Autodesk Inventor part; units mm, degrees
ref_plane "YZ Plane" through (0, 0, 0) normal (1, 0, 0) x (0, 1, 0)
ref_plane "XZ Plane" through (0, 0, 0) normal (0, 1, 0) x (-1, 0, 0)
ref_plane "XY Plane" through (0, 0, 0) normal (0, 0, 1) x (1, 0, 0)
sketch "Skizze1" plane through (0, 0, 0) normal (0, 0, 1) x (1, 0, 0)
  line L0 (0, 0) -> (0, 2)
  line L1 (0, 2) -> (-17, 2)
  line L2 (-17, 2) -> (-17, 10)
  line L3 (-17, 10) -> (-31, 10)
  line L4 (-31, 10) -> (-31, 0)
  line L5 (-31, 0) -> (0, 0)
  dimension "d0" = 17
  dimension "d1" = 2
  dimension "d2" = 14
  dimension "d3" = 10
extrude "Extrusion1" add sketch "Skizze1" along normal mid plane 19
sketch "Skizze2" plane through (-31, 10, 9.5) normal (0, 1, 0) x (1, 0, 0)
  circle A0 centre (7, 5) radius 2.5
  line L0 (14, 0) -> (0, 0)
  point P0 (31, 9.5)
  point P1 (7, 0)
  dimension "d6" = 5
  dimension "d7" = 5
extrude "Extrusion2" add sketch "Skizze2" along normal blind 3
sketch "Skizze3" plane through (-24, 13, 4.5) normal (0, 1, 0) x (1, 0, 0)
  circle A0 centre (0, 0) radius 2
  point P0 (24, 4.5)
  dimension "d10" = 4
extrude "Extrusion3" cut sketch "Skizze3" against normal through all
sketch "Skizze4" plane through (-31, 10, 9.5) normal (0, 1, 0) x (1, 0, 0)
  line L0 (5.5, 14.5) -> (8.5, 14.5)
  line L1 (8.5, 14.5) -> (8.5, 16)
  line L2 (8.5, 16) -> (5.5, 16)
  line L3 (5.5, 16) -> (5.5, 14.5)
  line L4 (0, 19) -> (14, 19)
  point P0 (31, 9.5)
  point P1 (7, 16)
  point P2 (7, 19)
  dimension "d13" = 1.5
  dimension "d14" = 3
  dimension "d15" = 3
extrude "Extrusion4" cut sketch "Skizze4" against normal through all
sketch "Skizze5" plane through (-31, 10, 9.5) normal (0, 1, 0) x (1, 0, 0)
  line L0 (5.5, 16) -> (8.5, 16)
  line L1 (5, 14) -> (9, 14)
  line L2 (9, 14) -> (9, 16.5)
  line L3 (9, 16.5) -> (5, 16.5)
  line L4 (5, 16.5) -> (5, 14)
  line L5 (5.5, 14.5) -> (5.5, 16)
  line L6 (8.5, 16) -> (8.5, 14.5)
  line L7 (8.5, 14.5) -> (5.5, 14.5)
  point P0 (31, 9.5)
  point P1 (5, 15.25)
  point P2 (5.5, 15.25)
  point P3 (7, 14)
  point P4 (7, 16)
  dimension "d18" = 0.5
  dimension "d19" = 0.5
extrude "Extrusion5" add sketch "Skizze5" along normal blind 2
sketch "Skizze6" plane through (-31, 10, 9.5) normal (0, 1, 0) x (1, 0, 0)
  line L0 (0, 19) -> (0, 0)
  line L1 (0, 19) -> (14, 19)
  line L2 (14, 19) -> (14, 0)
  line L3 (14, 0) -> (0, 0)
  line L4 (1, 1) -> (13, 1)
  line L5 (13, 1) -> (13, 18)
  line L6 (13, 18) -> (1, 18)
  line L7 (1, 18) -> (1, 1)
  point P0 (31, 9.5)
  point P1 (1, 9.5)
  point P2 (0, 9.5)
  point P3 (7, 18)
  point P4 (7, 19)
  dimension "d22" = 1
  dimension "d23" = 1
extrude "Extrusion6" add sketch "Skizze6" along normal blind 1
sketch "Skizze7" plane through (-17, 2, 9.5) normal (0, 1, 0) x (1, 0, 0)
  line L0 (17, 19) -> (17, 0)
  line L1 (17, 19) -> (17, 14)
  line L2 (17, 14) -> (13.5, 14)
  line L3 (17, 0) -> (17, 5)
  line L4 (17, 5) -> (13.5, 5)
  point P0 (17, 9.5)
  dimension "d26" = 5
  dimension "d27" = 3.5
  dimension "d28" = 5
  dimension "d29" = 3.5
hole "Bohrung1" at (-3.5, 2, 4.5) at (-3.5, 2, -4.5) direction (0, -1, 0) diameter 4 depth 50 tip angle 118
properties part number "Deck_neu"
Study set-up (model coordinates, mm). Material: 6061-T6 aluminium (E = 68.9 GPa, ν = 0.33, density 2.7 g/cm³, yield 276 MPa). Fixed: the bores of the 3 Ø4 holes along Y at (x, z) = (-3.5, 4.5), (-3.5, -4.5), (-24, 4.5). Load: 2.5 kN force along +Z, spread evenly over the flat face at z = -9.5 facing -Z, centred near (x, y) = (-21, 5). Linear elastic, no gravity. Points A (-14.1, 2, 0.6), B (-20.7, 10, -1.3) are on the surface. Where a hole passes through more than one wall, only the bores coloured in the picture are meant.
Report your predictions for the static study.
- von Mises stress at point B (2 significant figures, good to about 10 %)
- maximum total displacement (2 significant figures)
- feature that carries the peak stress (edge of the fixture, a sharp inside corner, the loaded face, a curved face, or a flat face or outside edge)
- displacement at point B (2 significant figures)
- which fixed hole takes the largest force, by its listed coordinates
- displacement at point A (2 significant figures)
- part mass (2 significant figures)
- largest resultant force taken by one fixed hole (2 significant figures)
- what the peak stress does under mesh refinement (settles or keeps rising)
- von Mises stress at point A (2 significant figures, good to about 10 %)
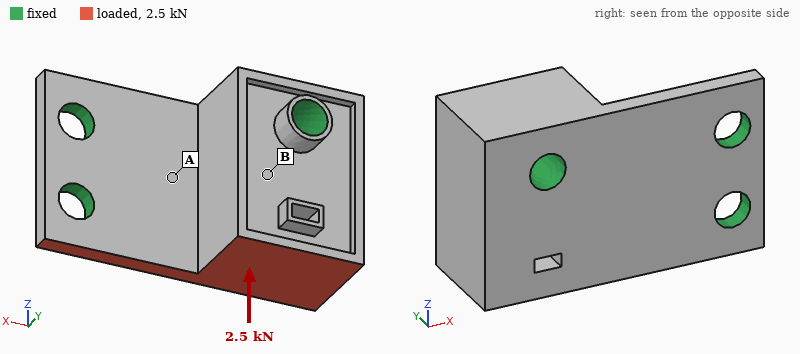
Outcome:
21 MPa
7.7 µm
a sharp inside corner
1.9 µm
(-24, 4.5)
1.6 µm
8.6 g
2.1 kN
keeps rising
6.0 MPa
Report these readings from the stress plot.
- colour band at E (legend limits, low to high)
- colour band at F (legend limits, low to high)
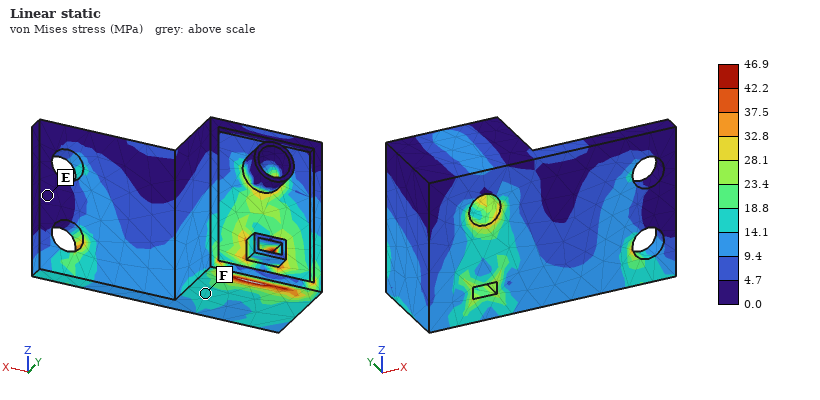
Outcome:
0.0 to 4.7 MPa
14.1 to 18.8 MPa
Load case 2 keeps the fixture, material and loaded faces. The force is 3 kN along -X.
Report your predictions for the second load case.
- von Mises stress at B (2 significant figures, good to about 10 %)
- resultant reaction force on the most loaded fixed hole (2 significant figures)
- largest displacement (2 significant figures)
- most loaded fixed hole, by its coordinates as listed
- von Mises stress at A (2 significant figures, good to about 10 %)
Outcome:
40 MPa
1.8 kN
38 µm
(-24, 4.5)
49 MPa
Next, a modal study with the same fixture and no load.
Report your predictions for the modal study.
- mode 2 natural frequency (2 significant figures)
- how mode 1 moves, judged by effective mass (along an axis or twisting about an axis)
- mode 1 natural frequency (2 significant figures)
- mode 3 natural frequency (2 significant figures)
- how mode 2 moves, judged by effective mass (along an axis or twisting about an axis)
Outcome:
33 kHz
along Y
30 kHz
45 kHz
along X
